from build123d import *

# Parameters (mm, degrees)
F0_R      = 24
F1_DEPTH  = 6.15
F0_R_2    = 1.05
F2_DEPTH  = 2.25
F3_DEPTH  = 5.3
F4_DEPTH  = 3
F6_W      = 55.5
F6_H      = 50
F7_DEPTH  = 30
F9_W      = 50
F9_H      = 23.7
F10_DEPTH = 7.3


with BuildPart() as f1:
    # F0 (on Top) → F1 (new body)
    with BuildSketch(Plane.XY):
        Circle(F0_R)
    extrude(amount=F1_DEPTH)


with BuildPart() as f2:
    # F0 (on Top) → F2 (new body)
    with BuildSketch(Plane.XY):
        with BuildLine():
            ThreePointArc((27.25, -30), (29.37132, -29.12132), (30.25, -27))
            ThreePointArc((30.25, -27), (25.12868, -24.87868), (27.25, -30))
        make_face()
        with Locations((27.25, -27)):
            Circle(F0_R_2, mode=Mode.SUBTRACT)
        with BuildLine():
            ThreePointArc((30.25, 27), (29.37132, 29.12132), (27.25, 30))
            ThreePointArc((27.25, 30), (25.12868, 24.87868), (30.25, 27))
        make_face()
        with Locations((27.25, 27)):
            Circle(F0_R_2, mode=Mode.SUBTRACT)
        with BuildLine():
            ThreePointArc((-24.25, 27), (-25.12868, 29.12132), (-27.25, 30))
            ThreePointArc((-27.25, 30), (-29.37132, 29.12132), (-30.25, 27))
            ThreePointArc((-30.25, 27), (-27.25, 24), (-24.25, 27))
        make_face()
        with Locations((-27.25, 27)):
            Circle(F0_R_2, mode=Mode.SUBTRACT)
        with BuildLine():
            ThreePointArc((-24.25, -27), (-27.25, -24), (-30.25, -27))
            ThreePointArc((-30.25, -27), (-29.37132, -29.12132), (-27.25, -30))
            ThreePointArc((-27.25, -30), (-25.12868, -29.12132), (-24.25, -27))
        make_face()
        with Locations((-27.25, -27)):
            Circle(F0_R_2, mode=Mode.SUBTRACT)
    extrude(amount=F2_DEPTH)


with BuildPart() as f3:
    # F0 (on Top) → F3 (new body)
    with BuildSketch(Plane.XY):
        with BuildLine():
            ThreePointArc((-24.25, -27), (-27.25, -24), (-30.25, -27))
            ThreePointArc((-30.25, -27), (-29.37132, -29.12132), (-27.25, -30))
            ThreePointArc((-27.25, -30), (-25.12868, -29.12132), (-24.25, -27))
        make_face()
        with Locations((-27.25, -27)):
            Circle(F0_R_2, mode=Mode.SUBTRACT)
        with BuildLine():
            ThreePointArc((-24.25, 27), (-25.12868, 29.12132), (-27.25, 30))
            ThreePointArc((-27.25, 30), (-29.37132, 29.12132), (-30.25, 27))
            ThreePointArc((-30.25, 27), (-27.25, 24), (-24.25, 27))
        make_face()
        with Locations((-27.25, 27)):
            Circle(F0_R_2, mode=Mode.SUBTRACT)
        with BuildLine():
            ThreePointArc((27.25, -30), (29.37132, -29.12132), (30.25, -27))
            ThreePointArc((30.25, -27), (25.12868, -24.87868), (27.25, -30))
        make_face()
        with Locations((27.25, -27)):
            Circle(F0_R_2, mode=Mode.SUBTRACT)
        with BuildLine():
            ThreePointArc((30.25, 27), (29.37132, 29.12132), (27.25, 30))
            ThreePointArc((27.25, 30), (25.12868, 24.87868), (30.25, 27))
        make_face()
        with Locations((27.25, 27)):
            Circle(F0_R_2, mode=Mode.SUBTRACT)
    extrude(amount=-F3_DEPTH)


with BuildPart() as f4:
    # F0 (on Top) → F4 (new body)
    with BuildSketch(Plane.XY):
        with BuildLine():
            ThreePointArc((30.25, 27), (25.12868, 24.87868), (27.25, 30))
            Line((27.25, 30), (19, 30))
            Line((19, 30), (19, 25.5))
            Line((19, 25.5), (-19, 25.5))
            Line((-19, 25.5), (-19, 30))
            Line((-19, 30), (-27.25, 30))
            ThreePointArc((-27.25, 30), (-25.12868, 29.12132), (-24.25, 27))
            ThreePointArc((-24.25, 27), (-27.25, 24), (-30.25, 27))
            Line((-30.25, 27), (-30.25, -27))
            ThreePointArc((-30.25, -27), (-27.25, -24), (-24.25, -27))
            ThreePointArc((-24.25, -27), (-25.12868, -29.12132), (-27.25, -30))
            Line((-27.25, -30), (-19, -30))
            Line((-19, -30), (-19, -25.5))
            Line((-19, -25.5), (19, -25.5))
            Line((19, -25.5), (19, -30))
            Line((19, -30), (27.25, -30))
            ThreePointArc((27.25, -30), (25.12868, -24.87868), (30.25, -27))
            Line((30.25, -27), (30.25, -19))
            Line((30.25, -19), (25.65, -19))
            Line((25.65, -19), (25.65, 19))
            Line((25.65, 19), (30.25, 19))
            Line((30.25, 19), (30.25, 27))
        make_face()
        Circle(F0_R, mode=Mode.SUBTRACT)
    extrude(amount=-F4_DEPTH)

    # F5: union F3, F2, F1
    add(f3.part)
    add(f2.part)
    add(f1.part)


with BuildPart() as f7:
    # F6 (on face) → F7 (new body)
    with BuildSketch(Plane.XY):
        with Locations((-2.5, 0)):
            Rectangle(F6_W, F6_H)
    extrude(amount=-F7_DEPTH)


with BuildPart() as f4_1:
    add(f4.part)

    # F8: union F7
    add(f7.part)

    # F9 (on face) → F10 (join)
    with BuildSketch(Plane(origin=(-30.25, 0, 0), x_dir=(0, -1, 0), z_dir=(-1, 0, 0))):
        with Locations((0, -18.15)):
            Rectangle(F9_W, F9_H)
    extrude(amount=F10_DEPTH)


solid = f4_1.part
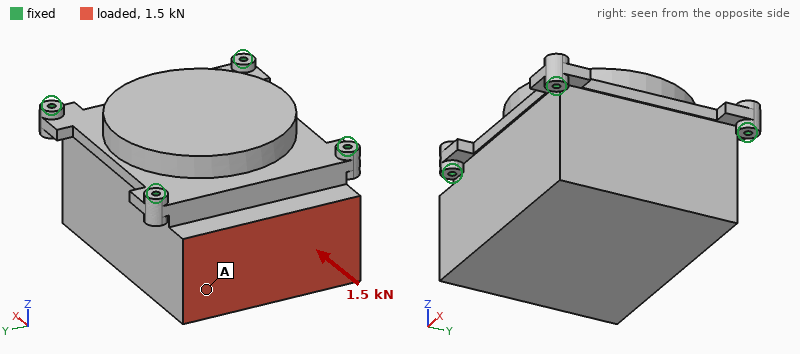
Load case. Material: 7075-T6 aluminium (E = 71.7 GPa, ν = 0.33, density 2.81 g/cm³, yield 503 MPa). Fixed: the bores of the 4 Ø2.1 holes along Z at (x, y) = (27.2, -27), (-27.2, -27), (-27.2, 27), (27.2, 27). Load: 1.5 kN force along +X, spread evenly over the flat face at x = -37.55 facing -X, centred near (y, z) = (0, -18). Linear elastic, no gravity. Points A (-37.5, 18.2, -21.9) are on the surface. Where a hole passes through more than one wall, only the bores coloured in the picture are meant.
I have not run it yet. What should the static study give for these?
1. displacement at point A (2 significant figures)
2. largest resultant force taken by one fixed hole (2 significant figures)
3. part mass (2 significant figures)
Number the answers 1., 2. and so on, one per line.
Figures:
1. 4.8 µm
2. 520 N
3. 290 g
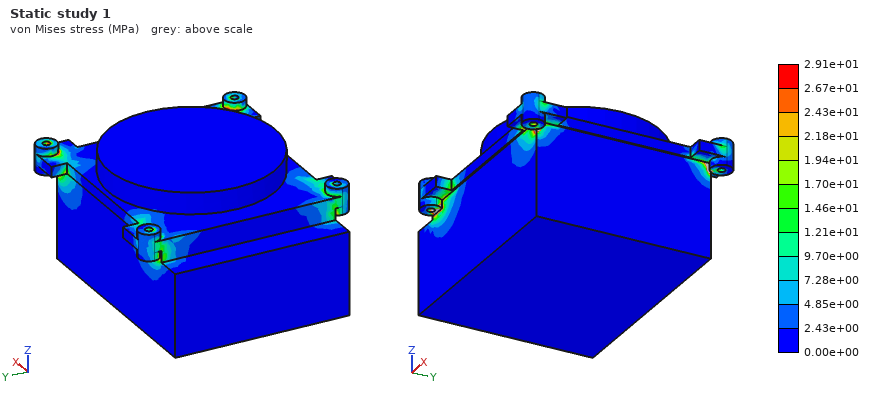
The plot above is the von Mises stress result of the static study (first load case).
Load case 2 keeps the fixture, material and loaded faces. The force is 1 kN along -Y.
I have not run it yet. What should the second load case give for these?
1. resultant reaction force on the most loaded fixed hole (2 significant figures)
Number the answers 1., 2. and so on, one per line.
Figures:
1. 560 N
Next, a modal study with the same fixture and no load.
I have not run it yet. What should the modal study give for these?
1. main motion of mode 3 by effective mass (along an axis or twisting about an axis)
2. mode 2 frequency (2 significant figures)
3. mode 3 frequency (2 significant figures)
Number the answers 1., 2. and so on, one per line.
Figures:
1. along Y
2. 6700 Hz
3. 7100 Hz
